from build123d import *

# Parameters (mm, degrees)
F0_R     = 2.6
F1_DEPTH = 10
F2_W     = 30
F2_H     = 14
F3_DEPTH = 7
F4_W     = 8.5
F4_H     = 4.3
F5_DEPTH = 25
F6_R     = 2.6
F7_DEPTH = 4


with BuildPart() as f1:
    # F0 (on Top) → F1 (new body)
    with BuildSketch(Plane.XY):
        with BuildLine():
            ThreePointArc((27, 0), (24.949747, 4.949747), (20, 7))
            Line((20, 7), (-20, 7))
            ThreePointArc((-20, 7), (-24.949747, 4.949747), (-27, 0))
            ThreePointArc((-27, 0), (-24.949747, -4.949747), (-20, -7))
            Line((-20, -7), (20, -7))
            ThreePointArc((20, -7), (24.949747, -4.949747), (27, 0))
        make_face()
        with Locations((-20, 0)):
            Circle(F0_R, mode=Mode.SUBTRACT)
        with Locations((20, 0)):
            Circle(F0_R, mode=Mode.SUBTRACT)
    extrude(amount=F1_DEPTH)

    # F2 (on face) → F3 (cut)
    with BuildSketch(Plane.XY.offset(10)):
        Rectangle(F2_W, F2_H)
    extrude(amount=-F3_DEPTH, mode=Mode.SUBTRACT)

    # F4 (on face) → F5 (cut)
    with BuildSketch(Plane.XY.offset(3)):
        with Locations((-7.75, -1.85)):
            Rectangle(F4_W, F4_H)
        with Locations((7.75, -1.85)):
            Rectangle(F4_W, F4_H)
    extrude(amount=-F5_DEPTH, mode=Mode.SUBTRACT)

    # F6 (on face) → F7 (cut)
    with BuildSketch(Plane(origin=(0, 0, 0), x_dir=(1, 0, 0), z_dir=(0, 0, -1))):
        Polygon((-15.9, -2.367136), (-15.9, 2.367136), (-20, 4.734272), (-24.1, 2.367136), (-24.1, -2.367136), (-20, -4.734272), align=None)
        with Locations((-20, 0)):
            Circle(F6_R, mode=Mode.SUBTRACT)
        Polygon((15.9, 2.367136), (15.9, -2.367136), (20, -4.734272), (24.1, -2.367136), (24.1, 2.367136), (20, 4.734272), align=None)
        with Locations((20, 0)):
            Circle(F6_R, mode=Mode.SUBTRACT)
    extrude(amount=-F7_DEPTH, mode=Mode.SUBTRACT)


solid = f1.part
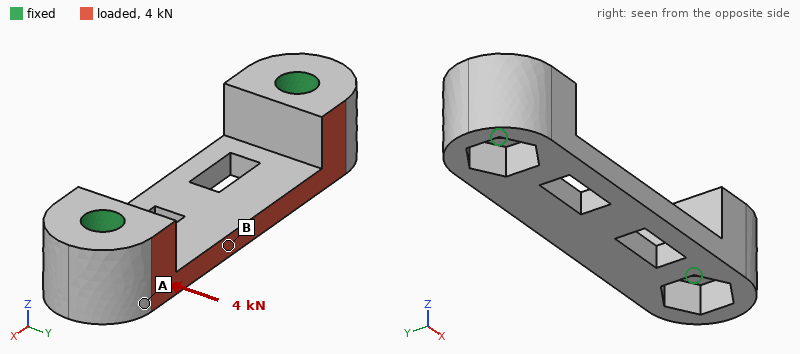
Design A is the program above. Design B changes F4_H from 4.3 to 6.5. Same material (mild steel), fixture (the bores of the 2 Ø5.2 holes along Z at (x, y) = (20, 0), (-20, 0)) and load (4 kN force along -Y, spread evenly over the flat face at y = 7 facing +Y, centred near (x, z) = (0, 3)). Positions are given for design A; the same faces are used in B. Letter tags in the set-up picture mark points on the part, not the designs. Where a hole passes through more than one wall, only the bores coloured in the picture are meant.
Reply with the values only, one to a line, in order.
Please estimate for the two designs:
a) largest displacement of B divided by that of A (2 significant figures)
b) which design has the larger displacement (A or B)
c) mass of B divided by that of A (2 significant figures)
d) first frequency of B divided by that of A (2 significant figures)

1.3
B
0.97
0.97
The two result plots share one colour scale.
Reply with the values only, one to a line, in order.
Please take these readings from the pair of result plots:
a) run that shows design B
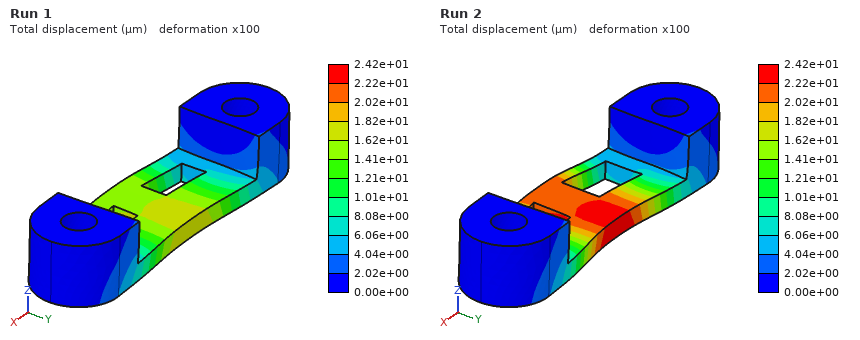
Run 2
